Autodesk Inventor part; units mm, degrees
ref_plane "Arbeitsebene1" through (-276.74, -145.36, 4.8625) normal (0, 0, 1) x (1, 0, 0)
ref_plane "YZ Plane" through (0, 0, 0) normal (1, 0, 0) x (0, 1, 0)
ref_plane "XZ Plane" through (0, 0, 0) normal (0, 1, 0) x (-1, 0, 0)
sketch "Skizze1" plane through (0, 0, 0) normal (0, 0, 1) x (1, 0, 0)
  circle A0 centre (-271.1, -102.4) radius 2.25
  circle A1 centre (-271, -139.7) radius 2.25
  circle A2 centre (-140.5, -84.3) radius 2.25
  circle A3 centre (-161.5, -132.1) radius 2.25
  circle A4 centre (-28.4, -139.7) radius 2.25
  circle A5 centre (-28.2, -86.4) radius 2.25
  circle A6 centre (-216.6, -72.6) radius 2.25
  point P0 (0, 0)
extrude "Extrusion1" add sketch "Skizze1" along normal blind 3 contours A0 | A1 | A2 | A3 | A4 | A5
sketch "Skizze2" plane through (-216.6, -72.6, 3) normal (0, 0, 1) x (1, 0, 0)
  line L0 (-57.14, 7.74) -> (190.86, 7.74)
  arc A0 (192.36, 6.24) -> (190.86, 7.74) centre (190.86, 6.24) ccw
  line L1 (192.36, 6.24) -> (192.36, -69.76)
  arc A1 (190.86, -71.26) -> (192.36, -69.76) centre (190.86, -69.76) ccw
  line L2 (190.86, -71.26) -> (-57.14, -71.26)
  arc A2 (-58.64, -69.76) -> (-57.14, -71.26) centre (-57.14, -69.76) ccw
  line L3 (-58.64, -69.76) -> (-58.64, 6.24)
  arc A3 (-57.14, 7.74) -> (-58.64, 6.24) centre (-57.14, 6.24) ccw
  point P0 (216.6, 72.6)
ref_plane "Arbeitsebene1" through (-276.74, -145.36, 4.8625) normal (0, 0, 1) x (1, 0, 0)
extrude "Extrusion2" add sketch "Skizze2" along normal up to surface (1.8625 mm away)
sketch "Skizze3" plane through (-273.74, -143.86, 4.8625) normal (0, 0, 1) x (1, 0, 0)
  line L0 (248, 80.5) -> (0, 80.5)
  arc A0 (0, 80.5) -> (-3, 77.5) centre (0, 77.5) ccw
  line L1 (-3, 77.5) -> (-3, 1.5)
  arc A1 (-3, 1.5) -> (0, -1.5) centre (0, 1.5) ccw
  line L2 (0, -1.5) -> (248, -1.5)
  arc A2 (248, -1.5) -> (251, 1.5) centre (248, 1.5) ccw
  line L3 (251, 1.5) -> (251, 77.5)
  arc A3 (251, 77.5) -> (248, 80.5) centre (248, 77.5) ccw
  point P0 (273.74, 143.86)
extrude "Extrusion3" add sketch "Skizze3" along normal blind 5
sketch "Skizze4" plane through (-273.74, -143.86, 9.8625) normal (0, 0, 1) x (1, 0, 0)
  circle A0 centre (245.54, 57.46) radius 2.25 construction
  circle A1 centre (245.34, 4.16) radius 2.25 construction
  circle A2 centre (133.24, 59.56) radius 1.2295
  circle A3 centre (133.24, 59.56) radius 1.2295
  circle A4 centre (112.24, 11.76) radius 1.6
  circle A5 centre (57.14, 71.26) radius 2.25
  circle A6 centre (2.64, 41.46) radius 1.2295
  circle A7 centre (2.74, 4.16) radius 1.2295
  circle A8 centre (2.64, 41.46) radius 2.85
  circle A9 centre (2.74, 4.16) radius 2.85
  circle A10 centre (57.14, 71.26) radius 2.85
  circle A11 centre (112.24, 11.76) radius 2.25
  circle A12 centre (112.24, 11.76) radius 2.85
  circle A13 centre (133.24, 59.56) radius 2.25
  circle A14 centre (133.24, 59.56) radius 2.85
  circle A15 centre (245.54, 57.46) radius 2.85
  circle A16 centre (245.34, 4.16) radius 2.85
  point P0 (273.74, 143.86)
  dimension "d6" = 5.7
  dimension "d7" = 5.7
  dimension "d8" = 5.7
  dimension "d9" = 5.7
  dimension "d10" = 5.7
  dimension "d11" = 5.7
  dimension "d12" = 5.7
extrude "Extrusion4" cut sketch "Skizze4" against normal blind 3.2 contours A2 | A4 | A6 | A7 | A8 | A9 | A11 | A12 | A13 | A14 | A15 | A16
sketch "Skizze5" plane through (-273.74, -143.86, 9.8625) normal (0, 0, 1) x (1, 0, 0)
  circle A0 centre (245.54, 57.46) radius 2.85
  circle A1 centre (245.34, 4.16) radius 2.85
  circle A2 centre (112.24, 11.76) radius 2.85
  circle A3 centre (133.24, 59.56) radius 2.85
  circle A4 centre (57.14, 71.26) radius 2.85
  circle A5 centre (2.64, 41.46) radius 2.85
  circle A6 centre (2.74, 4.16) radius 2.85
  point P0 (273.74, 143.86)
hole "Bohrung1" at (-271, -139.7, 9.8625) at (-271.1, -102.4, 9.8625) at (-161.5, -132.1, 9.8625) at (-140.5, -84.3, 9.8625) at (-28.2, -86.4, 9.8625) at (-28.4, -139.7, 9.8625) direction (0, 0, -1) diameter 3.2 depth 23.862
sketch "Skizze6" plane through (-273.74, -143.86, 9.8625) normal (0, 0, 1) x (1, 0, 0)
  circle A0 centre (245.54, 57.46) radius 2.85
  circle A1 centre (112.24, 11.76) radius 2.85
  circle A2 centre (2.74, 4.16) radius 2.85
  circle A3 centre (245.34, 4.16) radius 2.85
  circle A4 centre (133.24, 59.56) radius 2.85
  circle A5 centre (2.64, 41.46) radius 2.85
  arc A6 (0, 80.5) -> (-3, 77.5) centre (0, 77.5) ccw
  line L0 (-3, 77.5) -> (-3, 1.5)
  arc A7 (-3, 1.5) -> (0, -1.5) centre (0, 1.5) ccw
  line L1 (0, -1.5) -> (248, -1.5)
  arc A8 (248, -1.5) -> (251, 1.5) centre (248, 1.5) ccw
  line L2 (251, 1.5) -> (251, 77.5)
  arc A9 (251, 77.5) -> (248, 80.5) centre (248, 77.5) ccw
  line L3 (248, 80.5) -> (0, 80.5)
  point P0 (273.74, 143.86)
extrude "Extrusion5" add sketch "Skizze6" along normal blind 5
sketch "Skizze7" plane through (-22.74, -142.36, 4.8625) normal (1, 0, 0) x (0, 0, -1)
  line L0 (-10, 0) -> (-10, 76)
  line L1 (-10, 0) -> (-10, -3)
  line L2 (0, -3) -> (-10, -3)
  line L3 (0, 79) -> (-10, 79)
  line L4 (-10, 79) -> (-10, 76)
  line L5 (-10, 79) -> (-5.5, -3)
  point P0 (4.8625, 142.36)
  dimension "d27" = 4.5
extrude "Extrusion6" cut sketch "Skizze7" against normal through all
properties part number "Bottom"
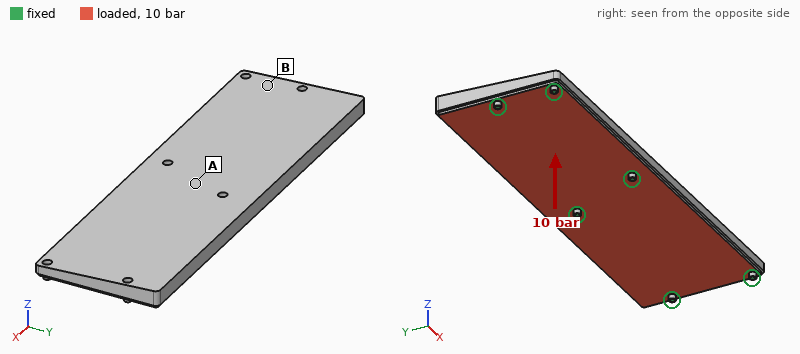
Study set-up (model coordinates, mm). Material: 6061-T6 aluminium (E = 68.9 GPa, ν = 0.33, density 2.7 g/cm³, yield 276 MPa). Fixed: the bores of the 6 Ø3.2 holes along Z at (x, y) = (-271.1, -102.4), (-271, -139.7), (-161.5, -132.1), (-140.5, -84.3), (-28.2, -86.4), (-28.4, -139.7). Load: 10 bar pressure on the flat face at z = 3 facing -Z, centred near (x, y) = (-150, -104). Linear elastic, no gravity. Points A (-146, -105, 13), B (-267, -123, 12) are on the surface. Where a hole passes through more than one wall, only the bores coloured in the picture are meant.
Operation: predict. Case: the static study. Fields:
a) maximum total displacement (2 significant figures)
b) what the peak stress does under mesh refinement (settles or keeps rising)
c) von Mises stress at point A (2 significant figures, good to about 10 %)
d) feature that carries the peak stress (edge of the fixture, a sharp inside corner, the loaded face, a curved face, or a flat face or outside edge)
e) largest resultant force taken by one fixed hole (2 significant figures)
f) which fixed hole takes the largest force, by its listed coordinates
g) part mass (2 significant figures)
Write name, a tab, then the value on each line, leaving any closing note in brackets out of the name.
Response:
maximum total displacement	0.28 mm
what the peak stress does under mesh refinement	keeps rising
von Mises stress at point A	69 MPa
feature that carries the peak stress	edge of the fixture
largest resultant force taken by one fixed hole	7.1 kN
which fixed hole takes the largest force, by its listed coordinates	(-140.5, -84.3)
part mass	530 g
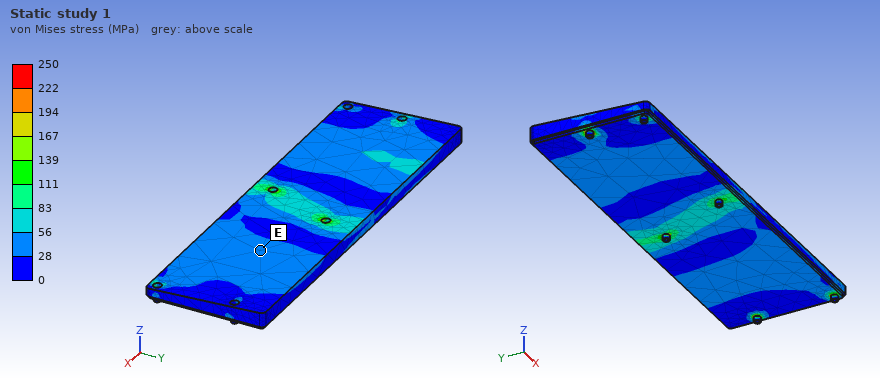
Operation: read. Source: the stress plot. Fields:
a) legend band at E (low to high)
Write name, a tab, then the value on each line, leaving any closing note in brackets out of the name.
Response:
legend band at E	28 to 56 MPa
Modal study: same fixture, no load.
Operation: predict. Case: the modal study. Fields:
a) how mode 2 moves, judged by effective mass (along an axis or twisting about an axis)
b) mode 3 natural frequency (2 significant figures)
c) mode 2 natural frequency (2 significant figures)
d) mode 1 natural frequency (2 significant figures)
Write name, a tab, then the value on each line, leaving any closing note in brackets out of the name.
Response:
how mode 2 moves, judged by effective mass	along Z
mode 3 natural frequency	3200 Hz
mode 2 natural frequency	2400 Hz
mode 1 natural frequency	1800 Hz
